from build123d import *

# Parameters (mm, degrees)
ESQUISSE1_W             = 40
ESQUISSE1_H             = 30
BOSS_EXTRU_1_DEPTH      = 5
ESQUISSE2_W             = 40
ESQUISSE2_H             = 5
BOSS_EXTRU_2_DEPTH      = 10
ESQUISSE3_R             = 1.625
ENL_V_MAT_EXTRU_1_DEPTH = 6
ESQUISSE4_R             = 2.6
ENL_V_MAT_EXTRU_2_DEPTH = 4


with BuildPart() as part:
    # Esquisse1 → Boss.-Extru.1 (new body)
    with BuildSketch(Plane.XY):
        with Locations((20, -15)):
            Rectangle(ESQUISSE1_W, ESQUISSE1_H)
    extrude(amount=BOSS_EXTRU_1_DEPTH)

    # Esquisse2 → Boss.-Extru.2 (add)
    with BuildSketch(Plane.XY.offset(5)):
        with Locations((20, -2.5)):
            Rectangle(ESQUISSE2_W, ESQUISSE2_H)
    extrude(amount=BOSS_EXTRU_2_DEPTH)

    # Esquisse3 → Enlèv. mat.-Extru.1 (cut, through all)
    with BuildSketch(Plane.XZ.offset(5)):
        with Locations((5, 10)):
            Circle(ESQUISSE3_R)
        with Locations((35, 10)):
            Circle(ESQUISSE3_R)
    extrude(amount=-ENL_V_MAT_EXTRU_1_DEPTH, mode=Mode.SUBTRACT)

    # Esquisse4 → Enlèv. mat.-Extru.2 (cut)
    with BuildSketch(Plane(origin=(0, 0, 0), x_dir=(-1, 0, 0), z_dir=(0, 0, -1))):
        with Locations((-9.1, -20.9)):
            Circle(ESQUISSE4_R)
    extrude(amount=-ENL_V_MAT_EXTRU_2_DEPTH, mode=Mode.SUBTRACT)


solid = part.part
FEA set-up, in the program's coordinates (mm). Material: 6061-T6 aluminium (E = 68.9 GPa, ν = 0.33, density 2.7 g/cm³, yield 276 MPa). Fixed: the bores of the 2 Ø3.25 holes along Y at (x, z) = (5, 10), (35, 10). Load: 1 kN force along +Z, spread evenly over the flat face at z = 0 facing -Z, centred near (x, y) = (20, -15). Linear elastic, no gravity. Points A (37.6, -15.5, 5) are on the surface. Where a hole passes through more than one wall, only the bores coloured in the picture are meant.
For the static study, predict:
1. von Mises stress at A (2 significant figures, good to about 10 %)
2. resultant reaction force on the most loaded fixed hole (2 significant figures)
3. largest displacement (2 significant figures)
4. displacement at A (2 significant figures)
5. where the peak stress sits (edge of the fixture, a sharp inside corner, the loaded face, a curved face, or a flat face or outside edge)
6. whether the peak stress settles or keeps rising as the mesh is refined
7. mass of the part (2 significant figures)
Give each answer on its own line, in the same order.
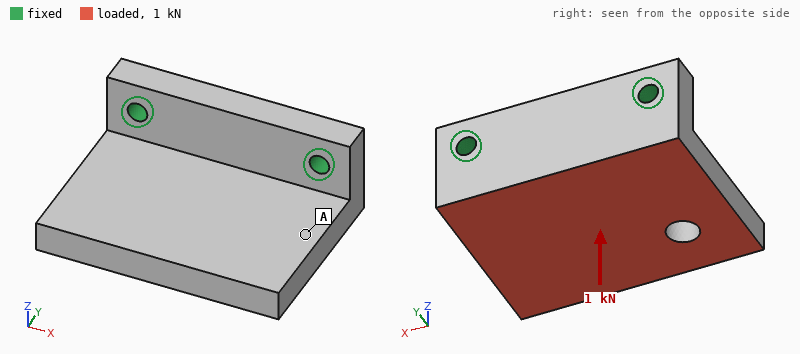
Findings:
19 MPa
530 N
0.18 mm
0.071 mm
edge of the fixture
keeps rising
21 g
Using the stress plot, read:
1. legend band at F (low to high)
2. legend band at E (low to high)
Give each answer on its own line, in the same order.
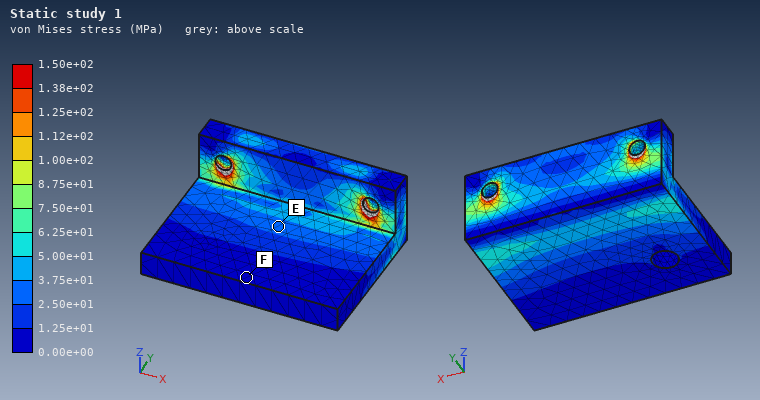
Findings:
0.00e+00 to 1.25e+01 MPa
2.50e+01 to 3.75e+01 MPa
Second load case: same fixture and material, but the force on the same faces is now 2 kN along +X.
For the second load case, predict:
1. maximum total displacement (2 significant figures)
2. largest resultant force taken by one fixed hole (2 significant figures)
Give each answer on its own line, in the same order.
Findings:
30 µm
1.4 kN
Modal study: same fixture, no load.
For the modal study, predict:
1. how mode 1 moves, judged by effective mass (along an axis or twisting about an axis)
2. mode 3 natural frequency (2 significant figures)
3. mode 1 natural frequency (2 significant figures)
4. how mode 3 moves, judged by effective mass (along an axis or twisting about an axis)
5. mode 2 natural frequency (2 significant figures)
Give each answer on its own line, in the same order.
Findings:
along Z
12 kHz
3600 Hz
along X
8000 Hz
